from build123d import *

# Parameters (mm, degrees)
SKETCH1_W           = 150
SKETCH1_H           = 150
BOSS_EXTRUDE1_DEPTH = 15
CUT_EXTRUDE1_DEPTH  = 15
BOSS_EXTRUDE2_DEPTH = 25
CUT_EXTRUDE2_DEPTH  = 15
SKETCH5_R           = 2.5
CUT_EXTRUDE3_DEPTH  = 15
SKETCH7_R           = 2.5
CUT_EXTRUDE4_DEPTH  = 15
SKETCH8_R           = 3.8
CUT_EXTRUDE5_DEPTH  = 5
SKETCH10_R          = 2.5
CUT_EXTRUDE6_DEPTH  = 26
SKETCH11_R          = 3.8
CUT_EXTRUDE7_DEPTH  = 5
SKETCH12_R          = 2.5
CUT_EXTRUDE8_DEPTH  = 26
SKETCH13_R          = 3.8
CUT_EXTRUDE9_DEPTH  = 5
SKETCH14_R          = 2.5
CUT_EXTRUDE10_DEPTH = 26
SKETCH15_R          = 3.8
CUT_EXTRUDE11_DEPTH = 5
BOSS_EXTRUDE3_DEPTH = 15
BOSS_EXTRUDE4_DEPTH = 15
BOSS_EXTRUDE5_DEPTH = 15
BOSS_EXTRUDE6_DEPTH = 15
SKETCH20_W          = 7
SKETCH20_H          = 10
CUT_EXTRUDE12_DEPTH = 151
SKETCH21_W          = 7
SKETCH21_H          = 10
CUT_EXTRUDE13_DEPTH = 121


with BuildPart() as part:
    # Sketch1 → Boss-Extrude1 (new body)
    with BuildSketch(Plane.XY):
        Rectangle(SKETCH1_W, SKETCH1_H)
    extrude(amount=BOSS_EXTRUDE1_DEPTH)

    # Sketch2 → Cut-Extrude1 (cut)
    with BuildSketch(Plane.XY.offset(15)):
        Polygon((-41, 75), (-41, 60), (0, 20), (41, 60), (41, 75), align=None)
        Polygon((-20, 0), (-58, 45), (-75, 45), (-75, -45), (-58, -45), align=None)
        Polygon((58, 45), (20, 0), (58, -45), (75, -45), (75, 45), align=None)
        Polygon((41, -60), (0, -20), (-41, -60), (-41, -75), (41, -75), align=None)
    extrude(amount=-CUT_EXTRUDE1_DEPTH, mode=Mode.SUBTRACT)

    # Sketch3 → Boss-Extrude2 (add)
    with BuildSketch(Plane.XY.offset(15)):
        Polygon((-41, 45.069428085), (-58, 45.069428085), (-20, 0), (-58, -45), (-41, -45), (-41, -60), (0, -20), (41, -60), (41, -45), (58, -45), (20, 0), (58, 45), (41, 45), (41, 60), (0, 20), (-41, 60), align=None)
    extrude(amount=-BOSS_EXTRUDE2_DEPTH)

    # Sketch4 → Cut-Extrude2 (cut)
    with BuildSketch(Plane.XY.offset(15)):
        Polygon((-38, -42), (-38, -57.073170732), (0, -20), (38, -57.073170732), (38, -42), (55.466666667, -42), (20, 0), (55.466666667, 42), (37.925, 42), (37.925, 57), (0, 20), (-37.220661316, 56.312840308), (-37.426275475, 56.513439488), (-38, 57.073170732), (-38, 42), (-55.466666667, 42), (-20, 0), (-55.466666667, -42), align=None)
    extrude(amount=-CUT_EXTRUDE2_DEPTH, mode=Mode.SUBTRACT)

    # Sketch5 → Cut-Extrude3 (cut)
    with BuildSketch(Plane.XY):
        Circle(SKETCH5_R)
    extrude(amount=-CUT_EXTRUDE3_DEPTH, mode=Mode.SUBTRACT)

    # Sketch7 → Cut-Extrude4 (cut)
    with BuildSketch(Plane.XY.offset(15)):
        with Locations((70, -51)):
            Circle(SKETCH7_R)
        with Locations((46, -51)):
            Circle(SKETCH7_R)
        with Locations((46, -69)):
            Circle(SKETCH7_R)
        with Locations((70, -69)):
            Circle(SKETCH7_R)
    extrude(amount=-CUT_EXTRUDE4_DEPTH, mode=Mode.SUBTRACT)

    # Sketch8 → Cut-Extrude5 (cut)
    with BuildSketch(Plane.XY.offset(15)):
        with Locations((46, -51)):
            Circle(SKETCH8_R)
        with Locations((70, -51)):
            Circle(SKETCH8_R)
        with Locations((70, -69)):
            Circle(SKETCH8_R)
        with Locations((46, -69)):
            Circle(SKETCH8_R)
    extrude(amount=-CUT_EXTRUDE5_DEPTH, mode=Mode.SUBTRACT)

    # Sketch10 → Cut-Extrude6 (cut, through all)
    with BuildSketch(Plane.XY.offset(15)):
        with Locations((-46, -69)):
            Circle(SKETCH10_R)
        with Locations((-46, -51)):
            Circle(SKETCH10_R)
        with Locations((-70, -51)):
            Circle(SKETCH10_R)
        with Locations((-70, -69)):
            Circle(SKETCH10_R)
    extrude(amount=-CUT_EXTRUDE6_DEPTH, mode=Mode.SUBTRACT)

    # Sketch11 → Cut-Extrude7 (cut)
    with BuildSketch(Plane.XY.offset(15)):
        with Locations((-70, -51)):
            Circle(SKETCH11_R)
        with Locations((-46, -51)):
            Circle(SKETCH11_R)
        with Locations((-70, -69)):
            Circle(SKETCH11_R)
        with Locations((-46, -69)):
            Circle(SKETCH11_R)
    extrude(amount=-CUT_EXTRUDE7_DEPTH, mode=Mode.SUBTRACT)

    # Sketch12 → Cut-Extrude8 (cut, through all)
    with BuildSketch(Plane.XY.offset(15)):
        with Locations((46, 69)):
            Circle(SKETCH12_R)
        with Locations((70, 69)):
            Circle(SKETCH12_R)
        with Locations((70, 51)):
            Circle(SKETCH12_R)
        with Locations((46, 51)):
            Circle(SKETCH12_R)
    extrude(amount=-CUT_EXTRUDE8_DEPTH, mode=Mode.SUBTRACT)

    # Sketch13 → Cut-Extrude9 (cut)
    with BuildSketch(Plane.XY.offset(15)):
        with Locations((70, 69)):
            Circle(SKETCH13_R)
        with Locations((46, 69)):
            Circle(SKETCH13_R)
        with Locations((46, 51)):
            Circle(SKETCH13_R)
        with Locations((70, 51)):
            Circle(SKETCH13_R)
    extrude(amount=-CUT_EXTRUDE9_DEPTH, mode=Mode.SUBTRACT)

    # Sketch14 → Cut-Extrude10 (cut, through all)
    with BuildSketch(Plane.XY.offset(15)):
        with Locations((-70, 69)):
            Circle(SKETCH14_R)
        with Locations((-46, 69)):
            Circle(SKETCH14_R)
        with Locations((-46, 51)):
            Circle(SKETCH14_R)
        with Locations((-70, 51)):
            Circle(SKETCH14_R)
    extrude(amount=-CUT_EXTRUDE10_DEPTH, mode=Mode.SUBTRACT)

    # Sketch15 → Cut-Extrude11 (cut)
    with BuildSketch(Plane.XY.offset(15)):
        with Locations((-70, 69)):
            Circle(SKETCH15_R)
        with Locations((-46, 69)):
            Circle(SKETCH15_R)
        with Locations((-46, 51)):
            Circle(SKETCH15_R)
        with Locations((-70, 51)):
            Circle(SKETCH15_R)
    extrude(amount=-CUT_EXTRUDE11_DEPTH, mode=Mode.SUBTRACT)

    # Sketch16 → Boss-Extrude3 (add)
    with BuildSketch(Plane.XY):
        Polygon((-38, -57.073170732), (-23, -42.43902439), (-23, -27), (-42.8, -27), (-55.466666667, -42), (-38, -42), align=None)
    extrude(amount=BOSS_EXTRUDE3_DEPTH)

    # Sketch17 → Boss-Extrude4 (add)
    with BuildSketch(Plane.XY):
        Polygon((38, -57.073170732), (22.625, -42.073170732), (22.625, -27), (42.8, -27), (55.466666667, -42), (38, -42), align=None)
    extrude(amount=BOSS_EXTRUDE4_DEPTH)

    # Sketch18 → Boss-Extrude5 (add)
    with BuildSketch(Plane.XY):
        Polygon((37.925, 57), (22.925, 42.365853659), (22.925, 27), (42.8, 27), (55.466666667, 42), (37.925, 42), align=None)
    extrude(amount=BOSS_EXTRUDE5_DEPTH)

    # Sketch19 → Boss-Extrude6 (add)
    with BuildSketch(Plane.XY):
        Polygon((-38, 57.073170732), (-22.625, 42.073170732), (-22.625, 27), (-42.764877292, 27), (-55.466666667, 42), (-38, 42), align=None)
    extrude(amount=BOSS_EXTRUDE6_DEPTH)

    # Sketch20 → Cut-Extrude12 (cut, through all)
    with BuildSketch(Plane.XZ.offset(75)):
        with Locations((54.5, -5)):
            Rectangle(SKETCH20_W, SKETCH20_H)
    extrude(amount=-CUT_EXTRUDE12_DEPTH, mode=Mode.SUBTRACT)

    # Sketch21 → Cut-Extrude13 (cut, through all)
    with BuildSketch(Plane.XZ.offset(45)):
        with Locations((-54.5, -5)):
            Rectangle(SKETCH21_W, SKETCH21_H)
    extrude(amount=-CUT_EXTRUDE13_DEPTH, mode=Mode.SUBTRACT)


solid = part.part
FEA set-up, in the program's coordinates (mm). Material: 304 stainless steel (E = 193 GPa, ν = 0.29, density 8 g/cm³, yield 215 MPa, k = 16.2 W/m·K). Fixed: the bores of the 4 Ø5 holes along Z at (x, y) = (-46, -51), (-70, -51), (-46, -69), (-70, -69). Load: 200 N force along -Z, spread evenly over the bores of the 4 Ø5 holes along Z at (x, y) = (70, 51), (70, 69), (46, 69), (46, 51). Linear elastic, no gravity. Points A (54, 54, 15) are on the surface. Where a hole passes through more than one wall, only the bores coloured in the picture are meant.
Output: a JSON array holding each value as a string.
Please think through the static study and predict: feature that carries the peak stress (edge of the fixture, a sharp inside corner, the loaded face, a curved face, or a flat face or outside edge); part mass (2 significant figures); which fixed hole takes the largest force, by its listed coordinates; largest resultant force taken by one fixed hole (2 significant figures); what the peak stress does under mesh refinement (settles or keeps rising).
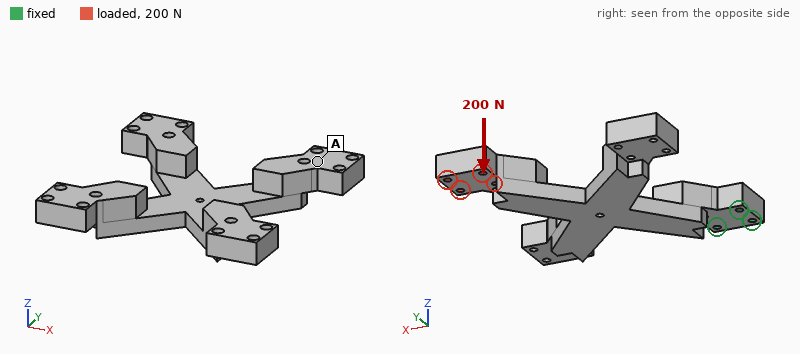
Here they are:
["edge of the fixture", "1.2 kg", "(-46, -51)", "1.2 kN", "keeps rising"]
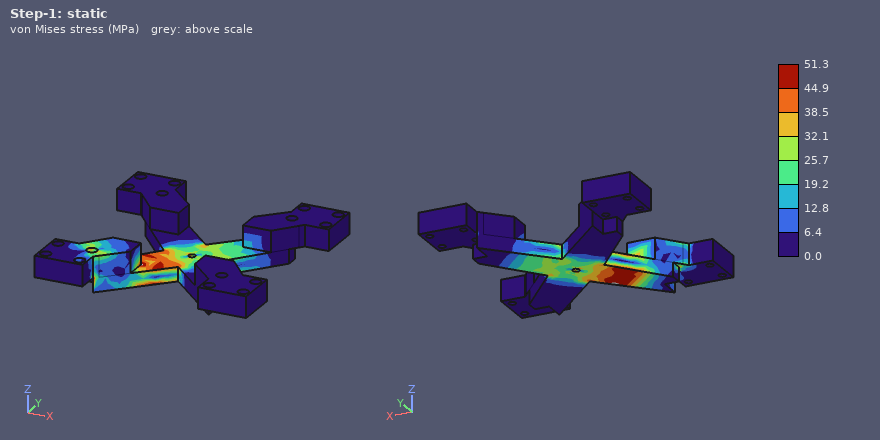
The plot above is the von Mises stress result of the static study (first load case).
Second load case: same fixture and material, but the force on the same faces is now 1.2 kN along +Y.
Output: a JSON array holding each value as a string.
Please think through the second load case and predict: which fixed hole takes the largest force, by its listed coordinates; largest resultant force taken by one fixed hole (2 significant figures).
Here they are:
["(-46, -51)", "3.0 kN"]
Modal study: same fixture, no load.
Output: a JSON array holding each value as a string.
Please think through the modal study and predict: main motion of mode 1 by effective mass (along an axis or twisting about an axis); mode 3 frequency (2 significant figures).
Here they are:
["along Z", "400 Hz"]
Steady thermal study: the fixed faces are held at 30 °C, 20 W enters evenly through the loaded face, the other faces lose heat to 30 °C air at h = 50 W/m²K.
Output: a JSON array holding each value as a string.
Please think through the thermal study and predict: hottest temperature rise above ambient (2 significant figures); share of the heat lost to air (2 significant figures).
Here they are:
["73 K", "99 %"]
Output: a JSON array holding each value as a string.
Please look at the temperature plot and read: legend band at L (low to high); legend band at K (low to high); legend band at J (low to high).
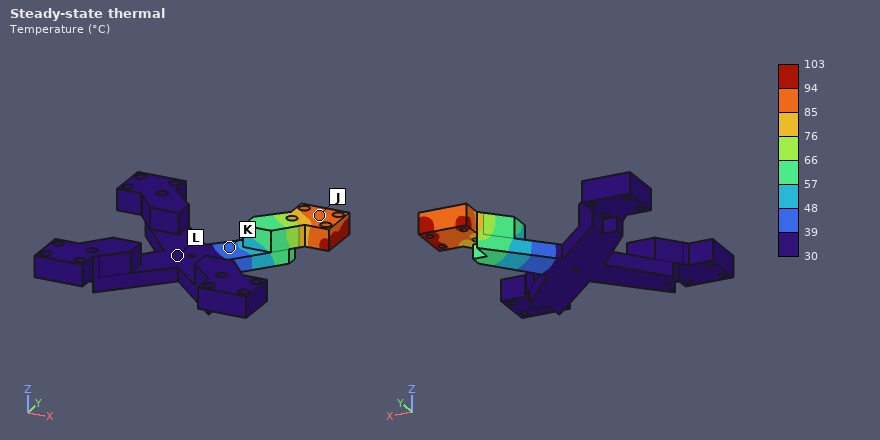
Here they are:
["30 to 39 °C", "39 to 48 °C", "85 to 94 °C"]
